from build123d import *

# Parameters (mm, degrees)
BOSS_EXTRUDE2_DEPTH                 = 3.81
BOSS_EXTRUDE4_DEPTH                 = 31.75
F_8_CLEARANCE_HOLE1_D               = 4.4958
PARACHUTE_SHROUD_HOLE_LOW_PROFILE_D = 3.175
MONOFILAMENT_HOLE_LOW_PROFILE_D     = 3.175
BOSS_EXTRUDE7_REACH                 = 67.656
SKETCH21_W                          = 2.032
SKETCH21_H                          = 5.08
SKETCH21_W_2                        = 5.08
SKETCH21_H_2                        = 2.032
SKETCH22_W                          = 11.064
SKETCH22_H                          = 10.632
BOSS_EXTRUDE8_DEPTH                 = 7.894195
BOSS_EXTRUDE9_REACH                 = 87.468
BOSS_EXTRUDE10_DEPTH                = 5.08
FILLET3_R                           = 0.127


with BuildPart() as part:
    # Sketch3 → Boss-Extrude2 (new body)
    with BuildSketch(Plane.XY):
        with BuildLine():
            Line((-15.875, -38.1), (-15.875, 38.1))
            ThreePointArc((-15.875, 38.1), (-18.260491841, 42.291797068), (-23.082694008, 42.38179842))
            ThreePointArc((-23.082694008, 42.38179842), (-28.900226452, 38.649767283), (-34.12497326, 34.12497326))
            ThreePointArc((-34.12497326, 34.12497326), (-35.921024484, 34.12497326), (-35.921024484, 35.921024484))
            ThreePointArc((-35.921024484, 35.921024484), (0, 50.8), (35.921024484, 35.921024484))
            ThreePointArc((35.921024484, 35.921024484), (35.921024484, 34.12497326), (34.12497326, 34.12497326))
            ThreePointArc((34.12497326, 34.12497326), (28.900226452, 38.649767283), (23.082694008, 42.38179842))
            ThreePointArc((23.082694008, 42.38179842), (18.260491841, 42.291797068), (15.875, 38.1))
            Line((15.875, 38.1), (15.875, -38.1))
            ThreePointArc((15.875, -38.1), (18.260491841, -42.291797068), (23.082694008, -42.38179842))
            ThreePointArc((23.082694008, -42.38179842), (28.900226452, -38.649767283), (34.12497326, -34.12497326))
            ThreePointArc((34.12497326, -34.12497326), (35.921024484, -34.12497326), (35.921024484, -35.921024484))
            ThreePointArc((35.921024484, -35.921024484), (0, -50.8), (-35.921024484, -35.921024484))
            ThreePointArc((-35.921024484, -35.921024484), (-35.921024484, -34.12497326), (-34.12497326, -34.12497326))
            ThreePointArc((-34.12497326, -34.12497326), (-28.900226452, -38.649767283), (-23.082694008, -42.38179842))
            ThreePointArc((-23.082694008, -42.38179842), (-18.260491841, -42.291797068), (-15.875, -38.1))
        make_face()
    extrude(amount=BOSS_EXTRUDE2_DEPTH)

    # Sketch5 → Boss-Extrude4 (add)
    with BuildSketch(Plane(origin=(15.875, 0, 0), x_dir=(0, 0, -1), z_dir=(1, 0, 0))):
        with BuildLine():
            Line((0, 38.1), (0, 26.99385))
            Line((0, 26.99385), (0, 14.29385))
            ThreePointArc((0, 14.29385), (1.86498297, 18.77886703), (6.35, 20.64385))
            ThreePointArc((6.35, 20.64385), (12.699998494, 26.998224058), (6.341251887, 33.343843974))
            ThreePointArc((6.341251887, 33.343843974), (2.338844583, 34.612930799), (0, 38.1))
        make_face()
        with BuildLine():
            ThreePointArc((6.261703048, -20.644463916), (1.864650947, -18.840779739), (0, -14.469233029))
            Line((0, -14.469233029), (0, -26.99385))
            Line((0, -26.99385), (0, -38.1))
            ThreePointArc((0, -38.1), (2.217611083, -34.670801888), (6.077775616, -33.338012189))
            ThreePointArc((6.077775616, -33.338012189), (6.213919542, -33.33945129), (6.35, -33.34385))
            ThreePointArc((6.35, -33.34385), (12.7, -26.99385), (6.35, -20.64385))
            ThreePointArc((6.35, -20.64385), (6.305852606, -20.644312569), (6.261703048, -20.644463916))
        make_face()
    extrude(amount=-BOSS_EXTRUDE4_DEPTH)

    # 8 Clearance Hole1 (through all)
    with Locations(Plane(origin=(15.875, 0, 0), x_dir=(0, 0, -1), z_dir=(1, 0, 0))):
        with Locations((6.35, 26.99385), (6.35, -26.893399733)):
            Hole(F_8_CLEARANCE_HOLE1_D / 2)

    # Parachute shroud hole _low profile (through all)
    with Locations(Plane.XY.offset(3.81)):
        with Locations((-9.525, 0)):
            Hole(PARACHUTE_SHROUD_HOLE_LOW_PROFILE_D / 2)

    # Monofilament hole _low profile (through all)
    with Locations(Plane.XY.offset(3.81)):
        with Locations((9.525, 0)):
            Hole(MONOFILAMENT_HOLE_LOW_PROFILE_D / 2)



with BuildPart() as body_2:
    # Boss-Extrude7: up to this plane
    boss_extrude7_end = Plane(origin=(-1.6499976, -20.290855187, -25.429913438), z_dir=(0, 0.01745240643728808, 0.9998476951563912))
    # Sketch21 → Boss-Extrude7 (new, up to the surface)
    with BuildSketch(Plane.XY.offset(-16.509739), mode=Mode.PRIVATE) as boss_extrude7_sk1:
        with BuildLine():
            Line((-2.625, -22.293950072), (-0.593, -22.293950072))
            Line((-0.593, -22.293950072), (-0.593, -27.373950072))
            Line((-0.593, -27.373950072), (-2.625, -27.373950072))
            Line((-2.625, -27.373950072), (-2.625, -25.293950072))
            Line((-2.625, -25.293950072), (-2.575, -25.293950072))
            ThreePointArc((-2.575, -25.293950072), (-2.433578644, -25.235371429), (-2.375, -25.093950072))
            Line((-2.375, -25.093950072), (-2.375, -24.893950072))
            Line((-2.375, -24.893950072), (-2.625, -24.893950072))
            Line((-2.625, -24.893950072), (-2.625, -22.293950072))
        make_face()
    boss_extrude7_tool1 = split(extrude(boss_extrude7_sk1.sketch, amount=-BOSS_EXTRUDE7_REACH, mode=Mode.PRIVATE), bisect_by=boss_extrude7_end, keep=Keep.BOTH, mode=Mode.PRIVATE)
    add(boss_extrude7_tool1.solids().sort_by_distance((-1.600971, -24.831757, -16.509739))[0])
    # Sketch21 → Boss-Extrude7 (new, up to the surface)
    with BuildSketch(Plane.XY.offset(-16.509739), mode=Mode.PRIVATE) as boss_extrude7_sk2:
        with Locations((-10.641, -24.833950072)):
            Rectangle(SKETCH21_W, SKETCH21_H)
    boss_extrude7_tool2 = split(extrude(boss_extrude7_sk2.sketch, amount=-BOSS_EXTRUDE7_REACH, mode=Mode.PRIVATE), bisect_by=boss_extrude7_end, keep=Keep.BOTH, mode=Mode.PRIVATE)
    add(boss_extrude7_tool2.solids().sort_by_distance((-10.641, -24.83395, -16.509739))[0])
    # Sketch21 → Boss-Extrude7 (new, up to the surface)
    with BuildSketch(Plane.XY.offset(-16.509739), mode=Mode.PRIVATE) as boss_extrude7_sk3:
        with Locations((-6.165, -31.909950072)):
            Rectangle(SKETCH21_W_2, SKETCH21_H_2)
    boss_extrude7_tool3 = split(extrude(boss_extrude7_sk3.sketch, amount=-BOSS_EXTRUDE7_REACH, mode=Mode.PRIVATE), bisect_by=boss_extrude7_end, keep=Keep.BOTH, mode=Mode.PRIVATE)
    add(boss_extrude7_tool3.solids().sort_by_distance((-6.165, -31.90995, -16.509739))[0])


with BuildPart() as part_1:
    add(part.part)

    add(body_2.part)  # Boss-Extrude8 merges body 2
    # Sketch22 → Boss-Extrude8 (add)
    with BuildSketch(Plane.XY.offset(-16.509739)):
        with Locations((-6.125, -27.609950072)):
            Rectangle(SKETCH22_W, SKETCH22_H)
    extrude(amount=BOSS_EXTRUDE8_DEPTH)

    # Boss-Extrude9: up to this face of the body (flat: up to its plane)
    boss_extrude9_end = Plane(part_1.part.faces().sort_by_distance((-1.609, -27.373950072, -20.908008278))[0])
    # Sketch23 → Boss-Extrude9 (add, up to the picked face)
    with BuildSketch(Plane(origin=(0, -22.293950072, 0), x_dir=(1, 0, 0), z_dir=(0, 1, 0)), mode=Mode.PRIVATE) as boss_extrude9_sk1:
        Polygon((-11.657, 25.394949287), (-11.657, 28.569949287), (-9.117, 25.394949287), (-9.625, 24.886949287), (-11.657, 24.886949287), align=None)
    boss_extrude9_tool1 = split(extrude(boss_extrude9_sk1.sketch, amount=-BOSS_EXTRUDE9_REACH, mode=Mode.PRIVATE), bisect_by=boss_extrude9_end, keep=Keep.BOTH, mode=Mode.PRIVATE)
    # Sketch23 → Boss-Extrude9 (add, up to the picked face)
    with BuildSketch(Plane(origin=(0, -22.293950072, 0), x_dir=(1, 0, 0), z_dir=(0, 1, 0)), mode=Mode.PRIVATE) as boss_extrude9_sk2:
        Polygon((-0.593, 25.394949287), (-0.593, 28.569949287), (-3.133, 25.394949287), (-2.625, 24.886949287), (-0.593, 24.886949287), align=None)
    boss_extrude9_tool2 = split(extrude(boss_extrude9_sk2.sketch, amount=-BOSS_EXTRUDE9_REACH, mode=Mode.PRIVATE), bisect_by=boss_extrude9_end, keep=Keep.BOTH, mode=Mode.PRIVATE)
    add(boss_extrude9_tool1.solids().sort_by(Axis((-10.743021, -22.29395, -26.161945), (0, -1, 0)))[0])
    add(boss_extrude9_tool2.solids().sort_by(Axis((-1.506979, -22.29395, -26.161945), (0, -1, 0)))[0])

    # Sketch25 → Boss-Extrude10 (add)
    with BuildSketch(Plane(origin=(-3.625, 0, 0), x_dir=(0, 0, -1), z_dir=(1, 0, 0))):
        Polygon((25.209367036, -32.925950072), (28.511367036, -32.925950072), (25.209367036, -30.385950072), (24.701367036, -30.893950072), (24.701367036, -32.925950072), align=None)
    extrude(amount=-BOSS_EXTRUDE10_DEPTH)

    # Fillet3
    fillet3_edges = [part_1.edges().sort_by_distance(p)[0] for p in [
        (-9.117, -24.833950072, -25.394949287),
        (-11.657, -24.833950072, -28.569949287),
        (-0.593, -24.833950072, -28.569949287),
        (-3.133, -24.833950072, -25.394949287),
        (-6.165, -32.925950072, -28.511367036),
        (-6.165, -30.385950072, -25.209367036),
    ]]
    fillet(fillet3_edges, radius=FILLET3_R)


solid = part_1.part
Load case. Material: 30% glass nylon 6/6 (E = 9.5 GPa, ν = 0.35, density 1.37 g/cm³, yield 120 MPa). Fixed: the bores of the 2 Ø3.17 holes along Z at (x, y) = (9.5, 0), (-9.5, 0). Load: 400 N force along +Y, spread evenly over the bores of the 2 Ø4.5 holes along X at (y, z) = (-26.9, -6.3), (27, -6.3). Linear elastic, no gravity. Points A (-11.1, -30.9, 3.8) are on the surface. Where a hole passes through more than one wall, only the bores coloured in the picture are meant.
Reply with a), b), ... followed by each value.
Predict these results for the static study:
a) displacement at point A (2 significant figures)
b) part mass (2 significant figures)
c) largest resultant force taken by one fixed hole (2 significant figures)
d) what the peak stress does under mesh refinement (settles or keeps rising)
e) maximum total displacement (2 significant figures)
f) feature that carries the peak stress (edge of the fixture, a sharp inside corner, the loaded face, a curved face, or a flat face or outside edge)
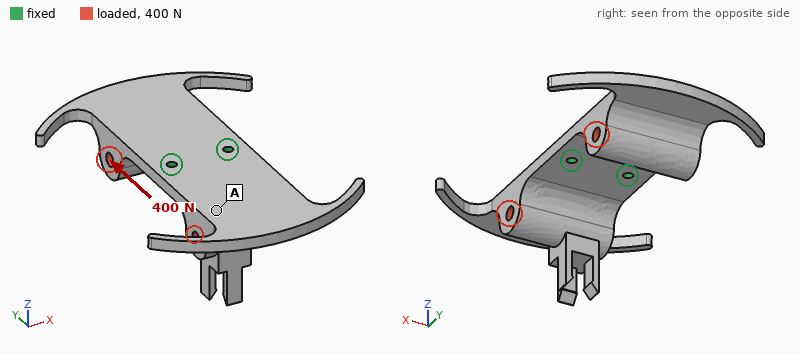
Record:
a) 0.49 mm
b) 32 g
c) 200 N
d) keeps rising
e) 0.93 mm
f) edge of the fixture
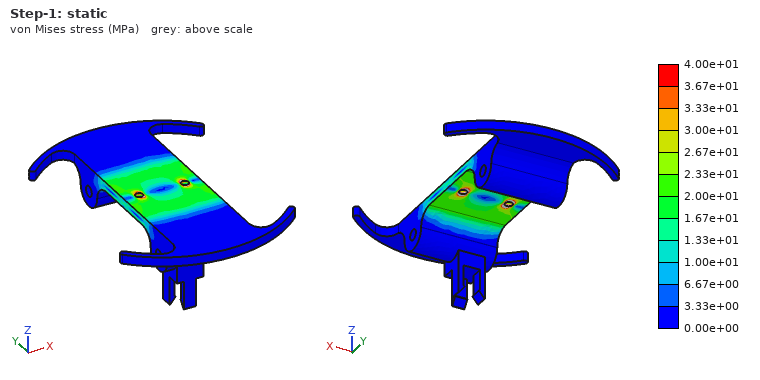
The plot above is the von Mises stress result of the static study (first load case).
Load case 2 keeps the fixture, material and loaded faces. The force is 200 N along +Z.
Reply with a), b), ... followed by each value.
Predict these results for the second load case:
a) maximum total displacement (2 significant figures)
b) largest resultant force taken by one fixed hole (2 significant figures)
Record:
a) 0.91 mm
b) 100 N
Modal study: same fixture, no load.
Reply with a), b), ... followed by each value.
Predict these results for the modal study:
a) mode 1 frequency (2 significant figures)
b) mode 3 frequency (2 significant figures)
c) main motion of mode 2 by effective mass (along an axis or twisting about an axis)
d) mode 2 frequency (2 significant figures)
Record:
a) 470 Hz
b) 1500 Hz
c) along Z
d) 530 Hz
